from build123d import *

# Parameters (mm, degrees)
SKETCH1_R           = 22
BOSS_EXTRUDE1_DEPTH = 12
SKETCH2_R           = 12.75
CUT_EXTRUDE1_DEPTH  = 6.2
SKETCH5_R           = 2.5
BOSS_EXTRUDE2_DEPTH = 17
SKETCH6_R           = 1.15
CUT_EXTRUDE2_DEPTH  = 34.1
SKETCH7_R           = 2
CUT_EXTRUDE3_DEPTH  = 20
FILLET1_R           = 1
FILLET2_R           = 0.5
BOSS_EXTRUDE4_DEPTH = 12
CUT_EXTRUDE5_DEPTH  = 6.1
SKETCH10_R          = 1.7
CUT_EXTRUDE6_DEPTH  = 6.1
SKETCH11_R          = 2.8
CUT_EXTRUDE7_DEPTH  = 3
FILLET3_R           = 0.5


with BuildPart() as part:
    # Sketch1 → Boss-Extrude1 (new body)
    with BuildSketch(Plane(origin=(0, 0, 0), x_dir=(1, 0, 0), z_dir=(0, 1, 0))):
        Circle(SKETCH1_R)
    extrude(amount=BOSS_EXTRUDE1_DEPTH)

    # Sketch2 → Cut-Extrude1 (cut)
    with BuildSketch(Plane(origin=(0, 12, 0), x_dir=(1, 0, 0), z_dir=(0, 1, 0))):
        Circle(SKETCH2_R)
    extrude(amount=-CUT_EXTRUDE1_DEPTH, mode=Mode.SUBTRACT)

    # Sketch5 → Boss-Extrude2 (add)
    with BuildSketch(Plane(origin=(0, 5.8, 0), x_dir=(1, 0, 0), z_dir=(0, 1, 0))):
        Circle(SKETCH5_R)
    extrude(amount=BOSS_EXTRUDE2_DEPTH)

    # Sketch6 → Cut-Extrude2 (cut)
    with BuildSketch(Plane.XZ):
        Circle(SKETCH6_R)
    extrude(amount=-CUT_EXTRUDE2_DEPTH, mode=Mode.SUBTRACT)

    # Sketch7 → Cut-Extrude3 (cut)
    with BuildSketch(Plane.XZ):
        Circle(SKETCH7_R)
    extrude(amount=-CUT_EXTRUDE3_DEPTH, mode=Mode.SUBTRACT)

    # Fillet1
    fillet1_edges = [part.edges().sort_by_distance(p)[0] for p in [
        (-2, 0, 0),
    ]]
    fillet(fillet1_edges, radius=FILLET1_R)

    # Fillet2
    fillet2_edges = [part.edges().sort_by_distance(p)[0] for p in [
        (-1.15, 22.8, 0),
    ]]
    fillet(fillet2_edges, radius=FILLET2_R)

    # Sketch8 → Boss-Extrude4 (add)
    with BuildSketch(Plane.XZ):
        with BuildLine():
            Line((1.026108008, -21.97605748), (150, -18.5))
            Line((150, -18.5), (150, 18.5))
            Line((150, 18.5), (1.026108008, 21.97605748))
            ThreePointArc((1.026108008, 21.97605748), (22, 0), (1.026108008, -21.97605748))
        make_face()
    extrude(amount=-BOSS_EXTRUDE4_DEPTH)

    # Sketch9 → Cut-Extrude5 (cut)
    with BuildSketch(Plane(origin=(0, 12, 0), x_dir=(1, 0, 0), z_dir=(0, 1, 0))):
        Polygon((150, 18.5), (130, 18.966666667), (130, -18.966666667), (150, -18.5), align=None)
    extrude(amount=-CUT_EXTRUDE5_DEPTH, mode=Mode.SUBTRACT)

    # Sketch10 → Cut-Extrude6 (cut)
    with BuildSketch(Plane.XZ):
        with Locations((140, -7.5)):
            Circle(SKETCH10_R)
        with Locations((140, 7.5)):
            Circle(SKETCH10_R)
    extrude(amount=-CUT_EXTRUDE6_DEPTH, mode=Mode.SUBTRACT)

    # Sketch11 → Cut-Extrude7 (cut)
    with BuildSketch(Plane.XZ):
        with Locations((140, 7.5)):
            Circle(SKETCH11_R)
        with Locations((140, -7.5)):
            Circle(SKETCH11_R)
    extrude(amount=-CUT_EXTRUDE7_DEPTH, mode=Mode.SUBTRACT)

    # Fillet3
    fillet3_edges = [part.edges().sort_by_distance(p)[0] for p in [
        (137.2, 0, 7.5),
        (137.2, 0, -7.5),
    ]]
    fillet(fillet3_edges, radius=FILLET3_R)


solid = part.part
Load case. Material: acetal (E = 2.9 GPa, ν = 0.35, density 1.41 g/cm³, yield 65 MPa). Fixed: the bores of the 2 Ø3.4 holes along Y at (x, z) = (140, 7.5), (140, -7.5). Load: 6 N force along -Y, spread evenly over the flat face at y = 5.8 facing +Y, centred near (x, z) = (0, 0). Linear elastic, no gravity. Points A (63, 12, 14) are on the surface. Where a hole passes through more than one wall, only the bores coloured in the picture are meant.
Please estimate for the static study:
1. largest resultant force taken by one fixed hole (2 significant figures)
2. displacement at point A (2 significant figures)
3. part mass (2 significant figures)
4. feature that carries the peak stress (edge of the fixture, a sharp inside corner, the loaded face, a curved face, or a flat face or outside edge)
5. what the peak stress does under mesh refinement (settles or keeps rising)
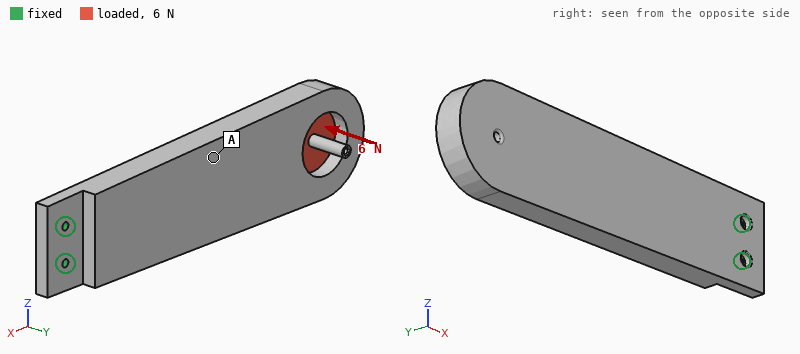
8.0 N
0.84 mm
100 g
edge of the fixture
keeps rising
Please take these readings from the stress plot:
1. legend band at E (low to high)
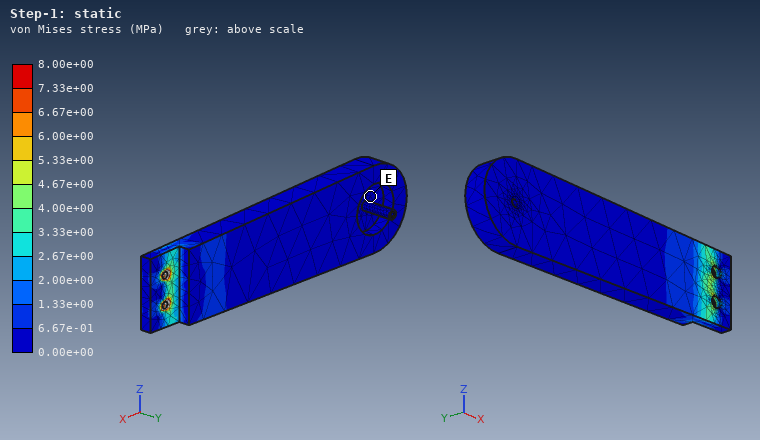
0.00e+00 to 6.67e-01 MPa
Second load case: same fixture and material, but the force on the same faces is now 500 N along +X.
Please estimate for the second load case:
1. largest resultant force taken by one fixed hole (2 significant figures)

250 N
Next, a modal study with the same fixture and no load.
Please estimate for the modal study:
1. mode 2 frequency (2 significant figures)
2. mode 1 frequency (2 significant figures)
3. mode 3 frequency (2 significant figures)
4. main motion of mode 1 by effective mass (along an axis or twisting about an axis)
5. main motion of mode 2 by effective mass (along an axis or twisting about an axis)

200 Hz
47 Hz
520 Hz
along Y
along Z
